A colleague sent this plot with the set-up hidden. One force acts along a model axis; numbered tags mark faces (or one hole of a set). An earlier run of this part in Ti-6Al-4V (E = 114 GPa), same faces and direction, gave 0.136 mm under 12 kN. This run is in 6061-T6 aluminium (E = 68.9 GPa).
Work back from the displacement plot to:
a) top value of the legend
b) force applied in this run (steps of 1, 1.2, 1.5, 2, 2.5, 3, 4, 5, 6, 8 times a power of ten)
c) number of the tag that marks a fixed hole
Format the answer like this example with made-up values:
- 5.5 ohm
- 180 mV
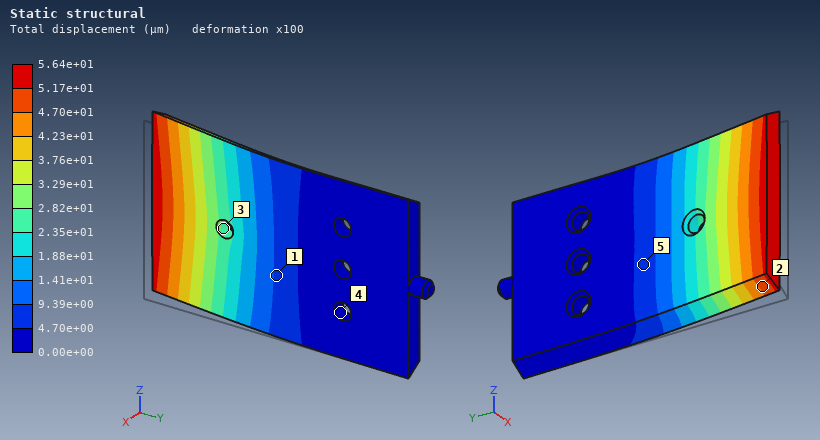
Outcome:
- 5.64e+01 µm
- 3 kN
- 4
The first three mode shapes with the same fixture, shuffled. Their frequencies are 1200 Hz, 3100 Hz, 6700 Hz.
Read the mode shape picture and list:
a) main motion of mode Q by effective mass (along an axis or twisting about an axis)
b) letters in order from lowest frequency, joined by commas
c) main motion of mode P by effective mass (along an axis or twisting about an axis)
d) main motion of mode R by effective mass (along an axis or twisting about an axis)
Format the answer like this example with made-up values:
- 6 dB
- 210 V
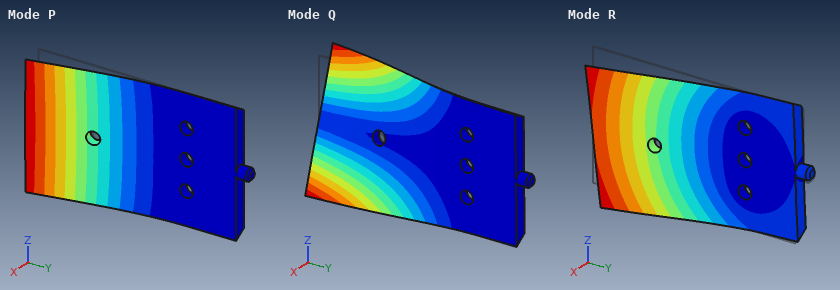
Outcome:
- twisting about Y
- P, Q, R
- along X
- along Z
